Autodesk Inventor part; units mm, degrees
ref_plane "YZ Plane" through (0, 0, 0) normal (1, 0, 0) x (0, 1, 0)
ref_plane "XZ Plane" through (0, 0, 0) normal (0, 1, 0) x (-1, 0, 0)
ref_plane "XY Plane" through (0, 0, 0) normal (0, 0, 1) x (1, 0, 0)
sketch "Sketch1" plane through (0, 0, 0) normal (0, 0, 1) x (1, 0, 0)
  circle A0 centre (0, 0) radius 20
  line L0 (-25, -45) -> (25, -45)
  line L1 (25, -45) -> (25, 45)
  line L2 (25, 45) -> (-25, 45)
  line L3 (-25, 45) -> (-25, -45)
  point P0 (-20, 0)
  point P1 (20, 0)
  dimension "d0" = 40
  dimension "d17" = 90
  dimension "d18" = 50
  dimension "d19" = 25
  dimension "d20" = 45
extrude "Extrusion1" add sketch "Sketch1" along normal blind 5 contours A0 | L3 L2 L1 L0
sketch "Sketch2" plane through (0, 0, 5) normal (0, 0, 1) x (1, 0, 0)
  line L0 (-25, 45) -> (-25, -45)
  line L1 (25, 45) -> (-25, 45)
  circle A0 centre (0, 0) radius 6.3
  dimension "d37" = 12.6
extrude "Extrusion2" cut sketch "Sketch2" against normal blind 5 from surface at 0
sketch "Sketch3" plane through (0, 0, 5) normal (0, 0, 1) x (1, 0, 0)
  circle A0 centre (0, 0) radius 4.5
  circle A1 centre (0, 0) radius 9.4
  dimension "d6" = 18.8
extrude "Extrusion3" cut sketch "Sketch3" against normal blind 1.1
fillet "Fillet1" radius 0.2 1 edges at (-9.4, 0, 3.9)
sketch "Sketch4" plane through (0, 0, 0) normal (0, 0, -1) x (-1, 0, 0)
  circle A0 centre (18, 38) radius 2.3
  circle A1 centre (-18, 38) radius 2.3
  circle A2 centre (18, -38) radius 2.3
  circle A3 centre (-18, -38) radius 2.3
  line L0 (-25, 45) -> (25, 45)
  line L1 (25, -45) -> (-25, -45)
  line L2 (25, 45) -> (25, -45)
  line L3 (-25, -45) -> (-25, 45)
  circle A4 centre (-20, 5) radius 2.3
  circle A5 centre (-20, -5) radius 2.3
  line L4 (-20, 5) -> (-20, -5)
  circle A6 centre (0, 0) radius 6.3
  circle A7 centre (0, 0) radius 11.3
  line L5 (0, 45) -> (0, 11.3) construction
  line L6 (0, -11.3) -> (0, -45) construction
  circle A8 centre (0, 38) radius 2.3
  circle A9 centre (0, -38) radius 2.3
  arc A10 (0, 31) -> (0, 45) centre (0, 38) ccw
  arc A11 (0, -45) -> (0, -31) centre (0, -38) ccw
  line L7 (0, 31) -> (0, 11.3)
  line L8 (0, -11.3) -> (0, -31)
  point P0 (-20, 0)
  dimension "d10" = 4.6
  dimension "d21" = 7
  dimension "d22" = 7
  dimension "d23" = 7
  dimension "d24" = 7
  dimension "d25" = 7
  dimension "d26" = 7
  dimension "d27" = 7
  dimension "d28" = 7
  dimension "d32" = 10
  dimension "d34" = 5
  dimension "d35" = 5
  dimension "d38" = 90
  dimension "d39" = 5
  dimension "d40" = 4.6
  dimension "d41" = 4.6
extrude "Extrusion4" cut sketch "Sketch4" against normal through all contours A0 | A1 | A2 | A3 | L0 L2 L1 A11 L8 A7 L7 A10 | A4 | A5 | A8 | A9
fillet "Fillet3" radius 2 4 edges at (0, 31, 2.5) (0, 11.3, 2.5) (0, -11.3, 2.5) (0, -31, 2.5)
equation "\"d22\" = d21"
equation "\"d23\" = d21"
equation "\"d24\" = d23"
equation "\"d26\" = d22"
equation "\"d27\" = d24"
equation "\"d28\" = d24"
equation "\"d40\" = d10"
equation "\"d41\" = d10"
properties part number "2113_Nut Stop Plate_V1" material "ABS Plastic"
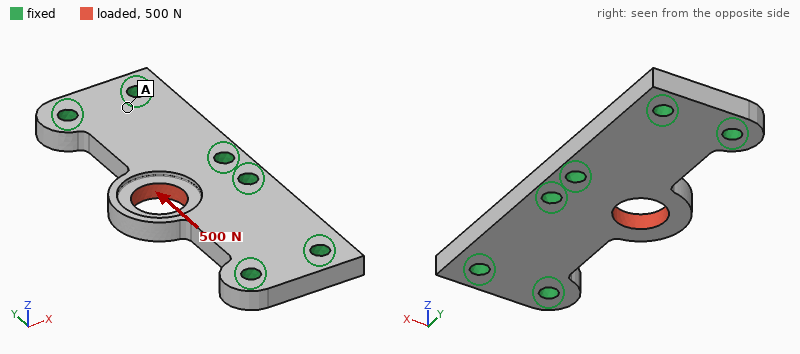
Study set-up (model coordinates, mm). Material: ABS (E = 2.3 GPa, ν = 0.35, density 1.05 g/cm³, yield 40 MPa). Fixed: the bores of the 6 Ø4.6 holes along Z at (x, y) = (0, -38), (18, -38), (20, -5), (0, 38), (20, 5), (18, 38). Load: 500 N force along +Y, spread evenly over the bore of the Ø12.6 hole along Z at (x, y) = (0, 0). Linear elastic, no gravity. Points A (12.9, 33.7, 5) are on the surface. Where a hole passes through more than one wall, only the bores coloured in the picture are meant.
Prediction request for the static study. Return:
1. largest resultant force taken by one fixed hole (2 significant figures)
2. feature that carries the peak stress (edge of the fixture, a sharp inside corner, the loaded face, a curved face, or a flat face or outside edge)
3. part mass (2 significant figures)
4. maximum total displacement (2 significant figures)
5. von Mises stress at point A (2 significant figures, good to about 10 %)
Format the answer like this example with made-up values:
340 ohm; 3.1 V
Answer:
130 N; a curved face; 12 g; 0.16 mm; 2.6 MPa
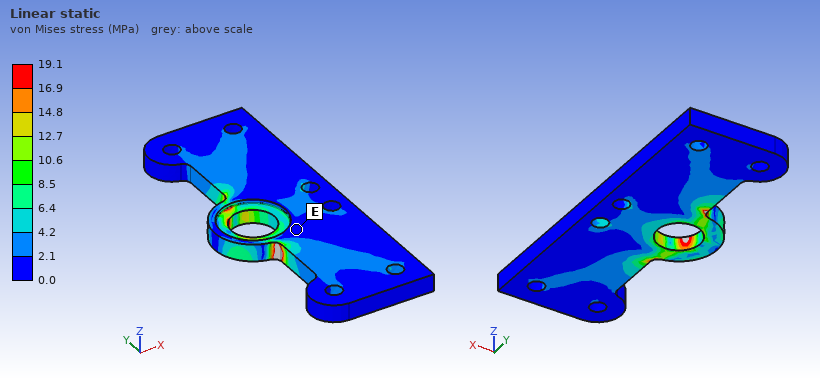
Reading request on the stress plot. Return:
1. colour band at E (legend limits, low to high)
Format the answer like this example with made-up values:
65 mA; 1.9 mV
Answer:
0.0 to 2.1 MPa
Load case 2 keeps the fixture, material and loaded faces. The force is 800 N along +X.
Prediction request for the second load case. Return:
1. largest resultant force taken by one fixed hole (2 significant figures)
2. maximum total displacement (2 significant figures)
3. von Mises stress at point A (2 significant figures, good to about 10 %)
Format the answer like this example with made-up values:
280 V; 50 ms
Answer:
330 N; 0.21 mm; 1.3 MPa
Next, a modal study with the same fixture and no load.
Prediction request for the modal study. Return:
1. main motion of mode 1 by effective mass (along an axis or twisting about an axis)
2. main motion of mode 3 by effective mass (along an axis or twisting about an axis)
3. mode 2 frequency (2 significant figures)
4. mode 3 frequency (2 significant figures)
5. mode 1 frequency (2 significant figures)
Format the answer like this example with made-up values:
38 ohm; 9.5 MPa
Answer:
along Z; along Z; 4300 Hz; 5500 Hz; 2200 Hz
